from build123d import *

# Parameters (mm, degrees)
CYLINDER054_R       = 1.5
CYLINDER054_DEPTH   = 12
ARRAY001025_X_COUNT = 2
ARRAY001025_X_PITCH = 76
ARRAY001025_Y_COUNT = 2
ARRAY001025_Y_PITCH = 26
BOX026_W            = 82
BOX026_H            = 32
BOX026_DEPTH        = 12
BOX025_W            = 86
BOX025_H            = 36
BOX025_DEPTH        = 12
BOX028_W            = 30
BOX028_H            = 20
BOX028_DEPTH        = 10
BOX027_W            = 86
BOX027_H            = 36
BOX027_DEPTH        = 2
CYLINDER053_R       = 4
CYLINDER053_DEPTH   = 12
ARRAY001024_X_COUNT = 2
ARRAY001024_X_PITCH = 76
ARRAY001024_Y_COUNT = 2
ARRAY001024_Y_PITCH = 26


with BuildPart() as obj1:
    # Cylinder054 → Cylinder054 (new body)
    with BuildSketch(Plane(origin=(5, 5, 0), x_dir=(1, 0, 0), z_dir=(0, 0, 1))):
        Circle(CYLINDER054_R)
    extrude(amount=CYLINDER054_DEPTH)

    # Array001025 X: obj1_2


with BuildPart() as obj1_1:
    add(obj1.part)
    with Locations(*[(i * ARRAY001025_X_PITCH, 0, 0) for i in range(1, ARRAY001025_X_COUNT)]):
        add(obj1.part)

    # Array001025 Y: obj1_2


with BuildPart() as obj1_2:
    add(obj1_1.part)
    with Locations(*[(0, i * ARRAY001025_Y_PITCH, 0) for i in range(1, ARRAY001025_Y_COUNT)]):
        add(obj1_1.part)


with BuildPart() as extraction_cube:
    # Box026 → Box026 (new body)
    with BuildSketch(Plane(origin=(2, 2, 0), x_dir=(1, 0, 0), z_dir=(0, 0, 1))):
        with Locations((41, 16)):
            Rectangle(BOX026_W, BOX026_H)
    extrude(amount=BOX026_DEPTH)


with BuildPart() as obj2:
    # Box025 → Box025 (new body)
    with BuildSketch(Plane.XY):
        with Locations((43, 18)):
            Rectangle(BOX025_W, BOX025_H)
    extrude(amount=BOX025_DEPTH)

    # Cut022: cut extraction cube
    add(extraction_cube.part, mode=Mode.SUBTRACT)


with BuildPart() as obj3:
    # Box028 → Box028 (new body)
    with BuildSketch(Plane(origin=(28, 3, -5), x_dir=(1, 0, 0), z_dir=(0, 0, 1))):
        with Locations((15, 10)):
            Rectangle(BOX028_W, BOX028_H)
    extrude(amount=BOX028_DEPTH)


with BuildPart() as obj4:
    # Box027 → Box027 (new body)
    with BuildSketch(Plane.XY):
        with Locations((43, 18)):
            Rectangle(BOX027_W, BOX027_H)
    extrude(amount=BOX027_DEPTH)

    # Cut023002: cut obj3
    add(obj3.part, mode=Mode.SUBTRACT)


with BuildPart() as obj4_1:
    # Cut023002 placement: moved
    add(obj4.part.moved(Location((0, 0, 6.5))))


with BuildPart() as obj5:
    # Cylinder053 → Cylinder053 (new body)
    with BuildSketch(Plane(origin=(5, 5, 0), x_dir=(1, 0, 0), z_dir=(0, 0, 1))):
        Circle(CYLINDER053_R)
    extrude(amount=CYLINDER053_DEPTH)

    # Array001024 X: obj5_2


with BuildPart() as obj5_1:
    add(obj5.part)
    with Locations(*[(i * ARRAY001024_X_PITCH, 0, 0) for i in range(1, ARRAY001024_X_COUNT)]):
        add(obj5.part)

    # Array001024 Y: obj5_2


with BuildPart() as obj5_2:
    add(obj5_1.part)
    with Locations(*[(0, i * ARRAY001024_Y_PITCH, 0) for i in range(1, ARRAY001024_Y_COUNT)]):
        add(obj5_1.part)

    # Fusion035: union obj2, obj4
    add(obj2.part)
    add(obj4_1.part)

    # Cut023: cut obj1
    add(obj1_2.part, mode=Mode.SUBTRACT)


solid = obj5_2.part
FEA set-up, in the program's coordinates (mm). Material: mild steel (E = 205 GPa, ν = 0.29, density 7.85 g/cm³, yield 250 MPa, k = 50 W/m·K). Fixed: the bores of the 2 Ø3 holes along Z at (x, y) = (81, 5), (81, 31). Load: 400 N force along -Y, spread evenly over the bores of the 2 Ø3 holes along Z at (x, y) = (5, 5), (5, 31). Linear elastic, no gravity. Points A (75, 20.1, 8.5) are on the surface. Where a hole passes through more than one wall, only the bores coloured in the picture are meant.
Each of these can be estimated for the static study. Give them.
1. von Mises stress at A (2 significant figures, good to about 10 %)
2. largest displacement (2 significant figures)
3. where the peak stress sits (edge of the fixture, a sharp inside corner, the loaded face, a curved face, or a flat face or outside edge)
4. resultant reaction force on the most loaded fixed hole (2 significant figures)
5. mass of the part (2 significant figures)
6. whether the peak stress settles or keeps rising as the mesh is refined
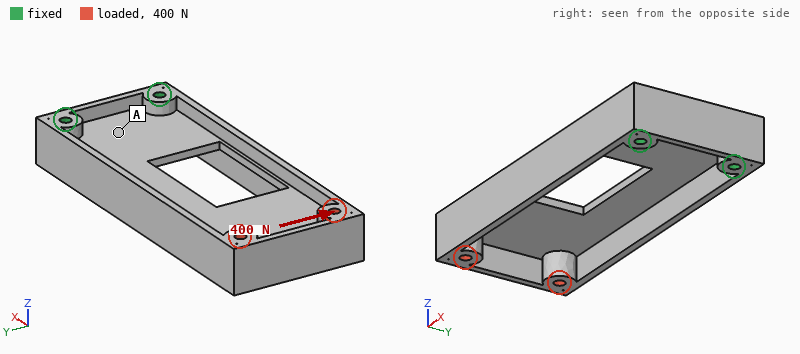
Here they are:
13 MPa
81 µm
a sharp inside corner
1.1 kN
87 g
keeps rising
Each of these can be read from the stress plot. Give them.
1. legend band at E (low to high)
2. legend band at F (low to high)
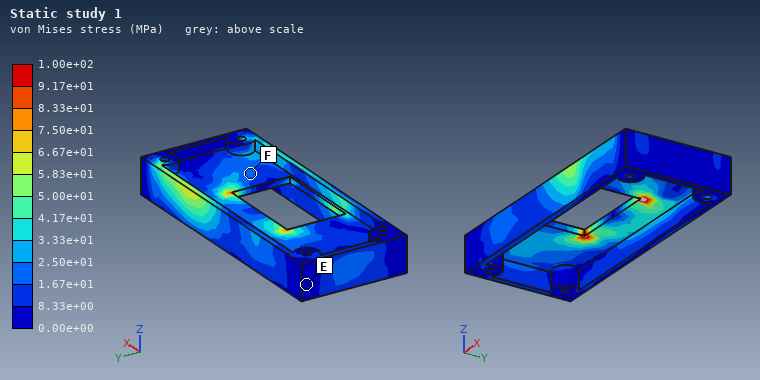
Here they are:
0.00e+00 to 8.33e+00 MPa
1.67e+01 to 2.50e+01 MPa
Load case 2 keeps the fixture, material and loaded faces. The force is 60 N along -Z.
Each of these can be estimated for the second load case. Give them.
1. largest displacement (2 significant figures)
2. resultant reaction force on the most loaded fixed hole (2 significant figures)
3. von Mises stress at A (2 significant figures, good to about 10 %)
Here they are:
78 µm
32 N
7.0 MPa
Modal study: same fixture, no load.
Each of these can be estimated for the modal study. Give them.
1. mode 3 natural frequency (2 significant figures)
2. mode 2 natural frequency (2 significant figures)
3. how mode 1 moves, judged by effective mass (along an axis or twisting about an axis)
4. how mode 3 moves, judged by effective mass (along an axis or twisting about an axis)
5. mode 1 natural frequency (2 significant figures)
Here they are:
2500 Hz
1500 Hz
along Z
along Y
830 Hz
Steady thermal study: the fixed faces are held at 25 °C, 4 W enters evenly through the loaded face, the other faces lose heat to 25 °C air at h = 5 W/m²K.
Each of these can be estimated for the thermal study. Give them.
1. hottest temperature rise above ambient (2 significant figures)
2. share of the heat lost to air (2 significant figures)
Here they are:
53 K
33 %
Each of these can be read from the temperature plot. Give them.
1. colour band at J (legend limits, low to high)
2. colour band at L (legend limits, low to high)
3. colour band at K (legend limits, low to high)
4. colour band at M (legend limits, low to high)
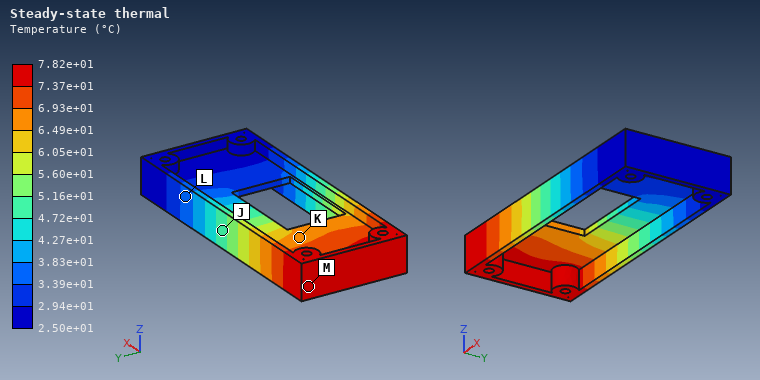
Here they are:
4.72e+01 to 5.16e+01 °C
3.39e+01 to 3.83e+01 °C
6.49e+01 to 6.93e+01 °C
7.37e+01 to 7.82e+01 °C
